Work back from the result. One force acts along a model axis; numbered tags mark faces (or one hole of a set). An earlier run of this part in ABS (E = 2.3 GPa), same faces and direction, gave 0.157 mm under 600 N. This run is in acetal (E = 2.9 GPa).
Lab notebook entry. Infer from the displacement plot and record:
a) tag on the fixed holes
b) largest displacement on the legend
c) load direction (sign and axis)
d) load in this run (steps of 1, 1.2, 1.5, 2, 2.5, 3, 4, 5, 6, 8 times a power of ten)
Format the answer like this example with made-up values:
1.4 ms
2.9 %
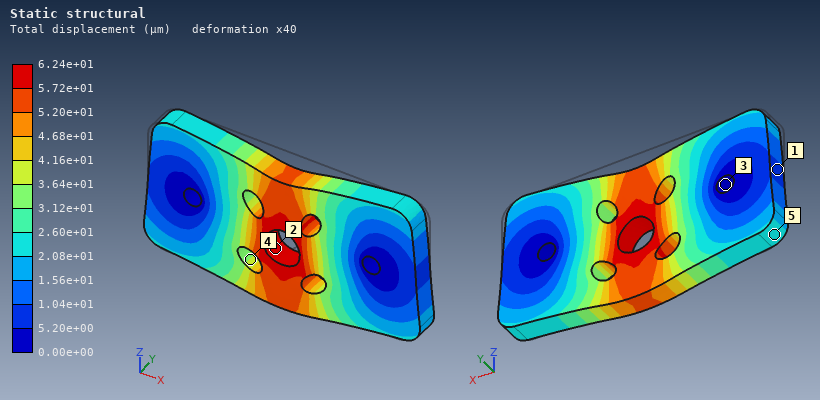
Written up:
3
6.24e+01 µm
-Z
300 N
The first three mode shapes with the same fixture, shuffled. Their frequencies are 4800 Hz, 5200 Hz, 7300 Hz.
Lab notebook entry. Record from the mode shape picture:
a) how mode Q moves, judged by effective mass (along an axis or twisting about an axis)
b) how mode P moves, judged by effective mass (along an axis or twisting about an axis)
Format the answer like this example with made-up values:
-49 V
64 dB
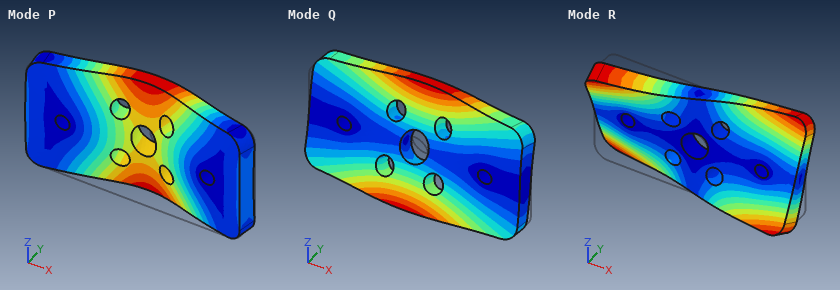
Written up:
twisting about X
along Y
